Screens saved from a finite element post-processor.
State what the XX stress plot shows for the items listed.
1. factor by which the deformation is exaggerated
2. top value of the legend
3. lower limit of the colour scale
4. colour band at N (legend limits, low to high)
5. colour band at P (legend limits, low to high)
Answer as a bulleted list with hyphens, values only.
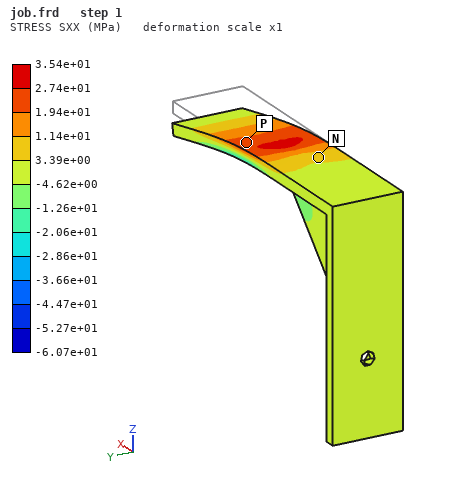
- 1
- 3.54e+01 MPa
- -6.07e+01 MPa
- 3.39e+00 to 1.14e+01 MPa
- 1.94e+01 to 2.74e+01 MPa
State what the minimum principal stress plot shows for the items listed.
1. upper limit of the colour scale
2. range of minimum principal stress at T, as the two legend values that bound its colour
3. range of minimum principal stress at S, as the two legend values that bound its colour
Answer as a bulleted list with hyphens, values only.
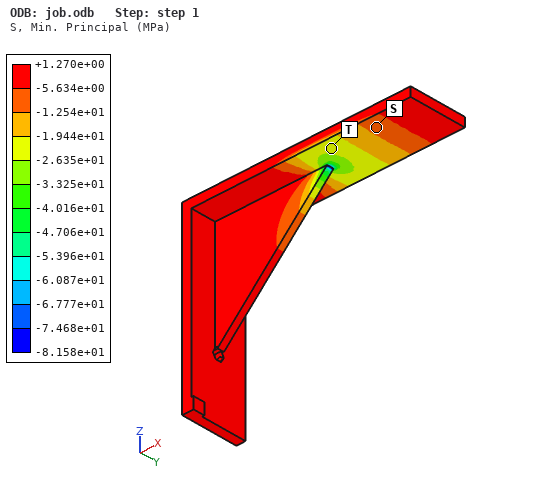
- +1.270e+00 MPa
- -2.635e+01 to -1.944e+01 MPa
- -1.254e+01 to -5.634e+00 MPa
